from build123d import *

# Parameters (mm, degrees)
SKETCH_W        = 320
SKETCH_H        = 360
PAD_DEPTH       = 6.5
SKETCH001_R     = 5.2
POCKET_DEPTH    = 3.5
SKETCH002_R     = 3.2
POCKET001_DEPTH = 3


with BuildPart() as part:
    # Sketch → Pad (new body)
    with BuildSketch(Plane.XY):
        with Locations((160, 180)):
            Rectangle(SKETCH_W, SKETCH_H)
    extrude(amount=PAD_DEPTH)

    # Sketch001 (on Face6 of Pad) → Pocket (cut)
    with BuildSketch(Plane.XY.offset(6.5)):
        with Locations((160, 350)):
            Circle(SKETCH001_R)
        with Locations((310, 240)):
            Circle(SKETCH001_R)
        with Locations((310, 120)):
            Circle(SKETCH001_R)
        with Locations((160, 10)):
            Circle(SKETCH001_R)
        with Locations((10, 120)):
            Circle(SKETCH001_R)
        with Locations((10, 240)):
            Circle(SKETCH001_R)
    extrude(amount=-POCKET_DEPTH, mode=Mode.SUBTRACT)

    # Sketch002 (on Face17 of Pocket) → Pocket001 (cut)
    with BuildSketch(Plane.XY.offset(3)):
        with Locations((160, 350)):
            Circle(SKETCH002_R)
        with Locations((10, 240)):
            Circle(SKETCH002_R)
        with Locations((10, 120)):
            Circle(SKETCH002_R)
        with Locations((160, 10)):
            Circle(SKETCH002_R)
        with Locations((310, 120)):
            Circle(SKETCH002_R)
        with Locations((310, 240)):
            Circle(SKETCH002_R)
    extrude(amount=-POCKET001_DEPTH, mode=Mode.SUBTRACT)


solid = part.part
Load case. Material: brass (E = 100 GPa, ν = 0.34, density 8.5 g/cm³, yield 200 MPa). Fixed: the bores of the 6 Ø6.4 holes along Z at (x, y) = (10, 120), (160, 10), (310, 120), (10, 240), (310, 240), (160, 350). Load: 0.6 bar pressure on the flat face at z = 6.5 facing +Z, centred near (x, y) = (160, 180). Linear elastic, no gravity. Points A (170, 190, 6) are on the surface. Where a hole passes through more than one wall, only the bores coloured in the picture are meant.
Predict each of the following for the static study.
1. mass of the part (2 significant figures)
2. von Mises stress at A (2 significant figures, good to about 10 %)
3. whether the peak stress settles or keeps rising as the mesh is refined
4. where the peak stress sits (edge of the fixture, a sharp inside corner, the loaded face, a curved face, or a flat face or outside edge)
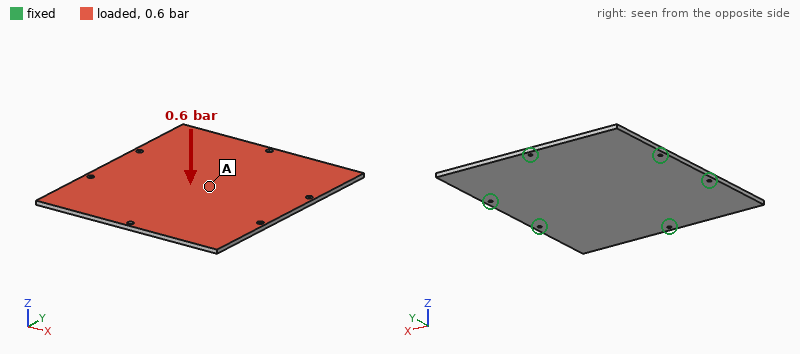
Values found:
6.3 kg
27 MPa
keeps rising
edge of the fixture
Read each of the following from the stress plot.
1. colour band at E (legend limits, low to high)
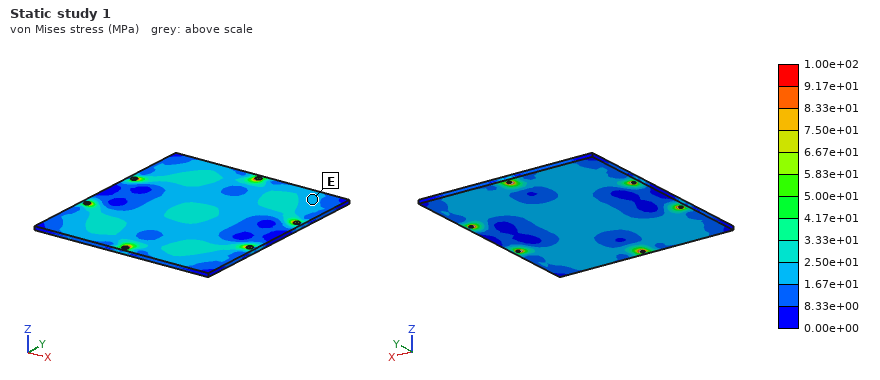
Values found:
1.67e+01 to 2.50e+01 MPa
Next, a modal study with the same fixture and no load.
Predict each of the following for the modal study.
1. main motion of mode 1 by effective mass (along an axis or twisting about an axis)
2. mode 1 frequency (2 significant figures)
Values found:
along Z
260 Hz
